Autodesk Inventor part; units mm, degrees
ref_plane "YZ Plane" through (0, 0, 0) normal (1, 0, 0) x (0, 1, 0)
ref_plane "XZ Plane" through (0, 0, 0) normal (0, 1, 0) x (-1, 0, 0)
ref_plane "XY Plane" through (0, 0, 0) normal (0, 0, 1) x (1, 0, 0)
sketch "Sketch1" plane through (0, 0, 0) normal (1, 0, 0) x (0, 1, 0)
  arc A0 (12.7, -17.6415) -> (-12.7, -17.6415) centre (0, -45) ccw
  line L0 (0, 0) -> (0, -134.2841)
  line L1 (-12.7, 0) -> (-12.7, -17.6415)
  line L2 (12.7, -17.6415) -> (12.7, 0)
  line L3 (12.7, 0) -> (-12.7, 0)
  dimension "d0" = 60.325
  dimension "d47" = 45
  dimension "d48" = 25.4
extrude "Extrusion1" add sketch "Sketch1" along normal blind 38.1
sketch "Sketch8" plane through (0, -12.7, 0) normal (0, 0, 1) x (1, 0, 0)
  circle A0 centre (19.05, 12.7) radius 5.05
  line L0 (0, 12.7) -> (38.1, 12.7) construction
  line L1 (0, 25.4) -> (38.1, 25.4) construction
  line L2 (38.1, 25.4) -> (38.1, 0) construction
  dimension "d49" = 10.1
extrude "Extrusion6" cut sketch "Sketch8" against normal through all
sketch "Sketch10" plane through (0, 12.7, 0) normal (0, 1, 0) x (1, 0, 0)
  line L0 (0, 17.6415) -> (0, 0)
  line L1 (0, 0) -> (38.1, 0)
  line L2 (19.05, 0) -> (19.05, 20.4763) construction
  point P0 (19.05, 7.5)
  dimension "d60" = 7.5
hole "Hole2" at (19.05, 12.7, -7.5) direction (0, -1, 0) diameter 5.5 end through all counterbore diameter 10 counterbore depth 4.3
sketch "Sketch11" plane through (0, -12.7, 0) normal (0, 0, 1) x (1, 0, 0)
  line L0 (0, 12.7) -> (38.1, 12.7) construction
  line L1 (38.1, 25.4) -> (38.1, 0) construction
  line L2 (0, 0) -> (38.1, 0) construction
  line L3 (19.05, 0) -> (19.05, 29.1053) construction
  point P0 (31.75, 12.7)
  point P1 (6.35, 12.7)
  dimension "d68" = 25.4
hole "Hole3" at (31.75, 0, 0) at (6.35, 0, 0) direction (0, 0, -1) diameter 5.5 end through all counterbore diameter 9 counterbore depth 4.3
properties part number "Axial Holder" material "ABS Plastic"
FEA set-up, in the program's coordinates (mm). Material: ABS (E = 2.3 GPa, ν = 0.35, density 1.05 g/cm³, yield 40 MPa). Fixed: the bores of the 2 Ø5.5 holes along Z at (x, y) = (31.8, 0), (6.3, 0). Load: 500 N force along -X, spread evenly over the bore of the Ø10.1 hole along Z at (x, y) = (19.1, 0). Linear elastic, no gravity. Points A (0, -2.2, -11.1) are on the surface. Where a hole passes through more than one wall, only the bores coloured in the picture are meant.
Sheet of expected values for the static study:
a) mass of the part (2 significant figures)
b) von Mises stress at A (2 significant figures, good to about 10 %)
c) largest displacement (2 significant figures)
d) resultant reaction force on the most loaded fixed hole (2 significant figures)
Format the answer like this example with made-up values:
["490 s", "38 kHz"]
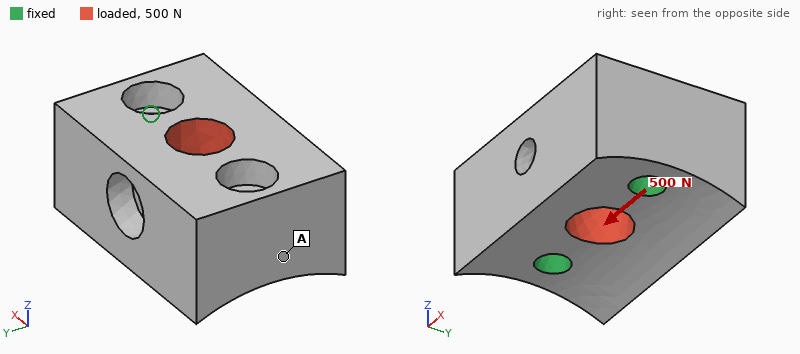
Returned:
["13 g", "0.73 MPa", "13 µm", "250 N"]
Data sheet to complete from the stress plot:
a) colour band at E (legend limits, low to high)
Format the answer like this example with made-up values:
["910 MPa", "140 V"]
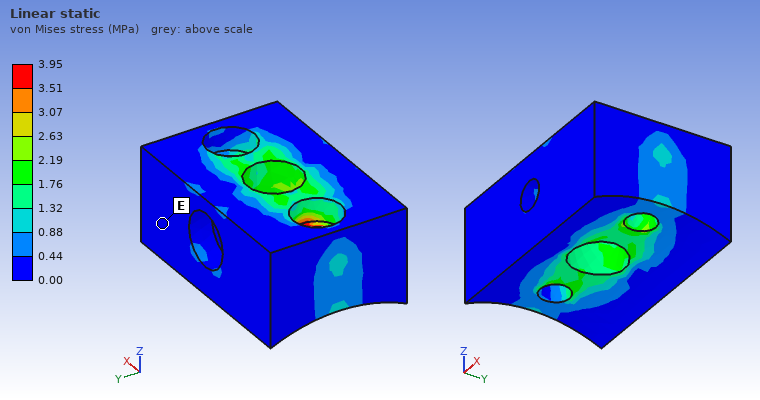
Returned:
["0.00 to 0.44 MPa"]
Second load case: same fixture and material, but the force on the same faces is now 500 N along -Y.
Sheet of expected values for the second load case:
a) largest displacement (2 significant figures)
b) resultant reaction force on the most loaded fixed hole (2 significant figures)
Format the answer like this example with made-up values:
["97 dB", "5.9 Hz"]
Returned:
["22 µm", "250 N"]
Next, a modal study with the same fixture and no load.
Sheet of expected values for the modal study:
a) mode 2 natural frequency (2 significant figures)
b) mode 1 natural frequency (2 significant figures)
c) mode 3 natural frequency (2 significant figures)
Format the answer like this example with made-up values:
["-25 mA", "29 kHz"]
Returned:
["10 kHz", "7900 Hz", "11 kHz"]
